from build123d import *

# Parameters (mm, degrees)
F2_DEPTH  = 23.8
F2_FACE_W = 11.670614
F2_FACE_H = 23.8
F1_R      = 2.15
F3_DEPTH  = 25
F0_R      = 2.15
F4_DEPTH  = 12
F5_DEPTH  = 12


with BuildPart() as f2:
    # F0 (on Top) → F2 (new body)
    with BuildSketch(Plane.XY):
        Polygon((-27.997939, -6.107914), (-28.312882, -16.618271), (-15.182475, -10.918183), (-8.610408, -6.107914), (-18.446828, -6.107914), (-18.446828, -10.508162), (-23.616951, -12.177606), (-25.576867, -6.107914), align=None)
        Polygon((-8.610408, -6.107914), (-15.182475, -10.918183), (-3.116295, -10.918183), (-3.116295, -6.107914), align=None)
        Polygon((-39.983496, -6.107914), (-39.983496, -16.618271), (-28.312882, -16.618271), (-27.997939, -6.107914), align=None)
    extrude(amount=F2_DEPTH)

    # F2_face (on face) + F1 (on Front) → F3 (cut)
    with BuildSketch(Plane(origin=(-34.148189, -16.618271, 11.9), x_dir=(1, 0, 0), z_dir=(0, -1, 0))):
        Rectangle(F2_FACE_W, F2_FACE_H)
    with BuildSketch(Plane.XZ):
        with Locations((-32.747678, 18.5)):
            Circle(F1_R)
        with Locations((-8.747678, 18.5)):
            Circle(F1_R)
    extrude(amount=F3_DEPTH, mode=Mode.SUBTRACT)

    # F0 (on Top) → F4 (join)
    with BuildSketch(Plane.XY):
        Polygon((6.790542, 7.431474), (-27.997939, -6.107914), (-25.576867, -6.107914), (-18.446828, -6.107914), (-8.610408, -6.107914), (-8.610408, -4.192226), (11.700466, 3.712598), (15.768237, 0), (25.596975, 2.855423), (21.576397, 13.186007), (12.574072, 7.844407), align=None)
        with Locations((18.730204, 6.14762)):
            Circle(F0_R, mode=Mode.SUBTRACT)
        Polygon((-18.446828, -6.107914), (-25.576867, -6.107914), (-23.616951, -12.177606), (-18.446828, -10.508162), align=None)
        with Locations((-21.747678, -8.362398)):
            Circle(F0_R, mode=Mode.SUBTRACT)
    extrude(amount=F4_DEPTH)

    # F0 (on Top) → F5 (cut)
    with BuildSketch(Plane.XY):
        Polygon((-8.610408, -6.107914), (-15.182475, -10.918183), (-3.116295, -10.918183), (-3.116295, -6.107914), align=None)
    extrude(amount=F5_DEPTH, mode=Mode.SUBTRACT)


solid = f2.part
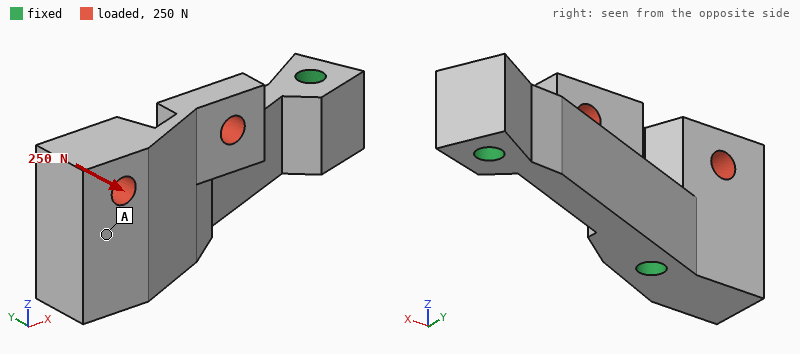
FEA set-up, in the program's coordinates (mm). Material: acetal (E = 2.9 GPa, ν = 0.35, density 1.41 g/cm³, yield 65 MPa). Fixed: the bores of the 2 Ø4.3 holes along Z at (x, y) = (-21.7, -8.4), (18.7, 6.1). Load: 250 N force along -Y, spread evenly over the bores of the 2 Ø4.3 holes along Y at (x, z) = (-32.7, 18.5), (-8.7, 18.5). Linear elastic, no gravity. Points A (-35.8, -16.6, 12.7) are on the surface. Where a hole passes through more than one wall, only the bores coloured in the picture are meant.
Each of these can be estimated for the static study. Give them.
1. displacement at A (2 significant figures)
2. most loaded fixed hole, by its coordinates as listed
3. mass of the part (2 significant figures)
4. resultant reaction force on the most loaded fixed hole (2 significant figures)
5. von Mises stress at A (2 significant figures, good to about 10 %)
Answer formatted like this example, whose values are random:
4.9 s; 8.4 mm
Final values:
0.11 mm; (-21.7, -8.4); 12 g; 250 N; 2.8 MPa
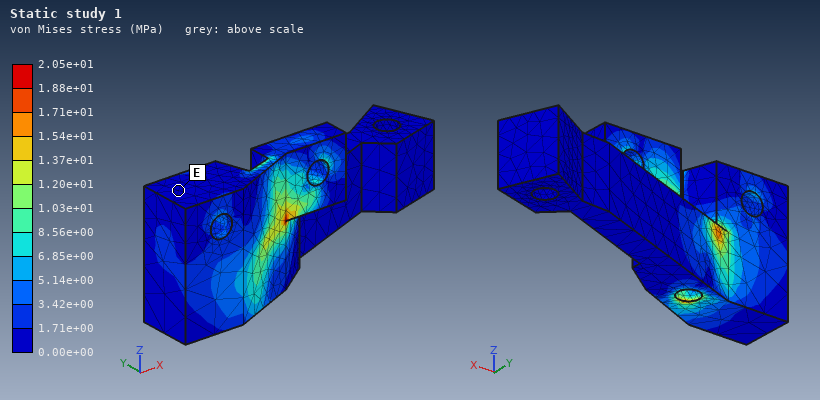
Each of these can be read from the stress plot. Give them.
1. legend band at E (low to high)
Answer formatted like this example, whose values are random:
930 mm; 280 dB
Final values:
0.00e+00 to 1.71e+00 MPa
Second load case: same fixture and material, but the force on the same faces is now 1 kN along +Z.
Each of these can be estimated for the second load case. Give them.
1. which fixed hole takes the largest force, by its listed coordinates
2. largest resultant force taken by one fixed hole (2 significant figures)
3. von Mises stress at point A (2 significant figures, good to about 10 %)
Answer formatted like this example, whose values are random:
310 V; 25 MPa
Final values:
(-21.7, -8.4); 990 N; 4.5 MPa
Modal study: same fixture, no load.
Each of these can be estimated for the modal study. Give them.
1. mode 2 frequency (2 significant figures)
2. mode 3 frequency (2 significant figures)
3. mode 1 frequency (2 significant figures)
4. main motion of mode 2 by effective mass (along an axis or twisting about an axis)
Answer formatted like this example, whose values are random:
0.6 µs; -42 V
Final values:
3200 Hz; 4300 Hz; 3100 Hz; along Y
